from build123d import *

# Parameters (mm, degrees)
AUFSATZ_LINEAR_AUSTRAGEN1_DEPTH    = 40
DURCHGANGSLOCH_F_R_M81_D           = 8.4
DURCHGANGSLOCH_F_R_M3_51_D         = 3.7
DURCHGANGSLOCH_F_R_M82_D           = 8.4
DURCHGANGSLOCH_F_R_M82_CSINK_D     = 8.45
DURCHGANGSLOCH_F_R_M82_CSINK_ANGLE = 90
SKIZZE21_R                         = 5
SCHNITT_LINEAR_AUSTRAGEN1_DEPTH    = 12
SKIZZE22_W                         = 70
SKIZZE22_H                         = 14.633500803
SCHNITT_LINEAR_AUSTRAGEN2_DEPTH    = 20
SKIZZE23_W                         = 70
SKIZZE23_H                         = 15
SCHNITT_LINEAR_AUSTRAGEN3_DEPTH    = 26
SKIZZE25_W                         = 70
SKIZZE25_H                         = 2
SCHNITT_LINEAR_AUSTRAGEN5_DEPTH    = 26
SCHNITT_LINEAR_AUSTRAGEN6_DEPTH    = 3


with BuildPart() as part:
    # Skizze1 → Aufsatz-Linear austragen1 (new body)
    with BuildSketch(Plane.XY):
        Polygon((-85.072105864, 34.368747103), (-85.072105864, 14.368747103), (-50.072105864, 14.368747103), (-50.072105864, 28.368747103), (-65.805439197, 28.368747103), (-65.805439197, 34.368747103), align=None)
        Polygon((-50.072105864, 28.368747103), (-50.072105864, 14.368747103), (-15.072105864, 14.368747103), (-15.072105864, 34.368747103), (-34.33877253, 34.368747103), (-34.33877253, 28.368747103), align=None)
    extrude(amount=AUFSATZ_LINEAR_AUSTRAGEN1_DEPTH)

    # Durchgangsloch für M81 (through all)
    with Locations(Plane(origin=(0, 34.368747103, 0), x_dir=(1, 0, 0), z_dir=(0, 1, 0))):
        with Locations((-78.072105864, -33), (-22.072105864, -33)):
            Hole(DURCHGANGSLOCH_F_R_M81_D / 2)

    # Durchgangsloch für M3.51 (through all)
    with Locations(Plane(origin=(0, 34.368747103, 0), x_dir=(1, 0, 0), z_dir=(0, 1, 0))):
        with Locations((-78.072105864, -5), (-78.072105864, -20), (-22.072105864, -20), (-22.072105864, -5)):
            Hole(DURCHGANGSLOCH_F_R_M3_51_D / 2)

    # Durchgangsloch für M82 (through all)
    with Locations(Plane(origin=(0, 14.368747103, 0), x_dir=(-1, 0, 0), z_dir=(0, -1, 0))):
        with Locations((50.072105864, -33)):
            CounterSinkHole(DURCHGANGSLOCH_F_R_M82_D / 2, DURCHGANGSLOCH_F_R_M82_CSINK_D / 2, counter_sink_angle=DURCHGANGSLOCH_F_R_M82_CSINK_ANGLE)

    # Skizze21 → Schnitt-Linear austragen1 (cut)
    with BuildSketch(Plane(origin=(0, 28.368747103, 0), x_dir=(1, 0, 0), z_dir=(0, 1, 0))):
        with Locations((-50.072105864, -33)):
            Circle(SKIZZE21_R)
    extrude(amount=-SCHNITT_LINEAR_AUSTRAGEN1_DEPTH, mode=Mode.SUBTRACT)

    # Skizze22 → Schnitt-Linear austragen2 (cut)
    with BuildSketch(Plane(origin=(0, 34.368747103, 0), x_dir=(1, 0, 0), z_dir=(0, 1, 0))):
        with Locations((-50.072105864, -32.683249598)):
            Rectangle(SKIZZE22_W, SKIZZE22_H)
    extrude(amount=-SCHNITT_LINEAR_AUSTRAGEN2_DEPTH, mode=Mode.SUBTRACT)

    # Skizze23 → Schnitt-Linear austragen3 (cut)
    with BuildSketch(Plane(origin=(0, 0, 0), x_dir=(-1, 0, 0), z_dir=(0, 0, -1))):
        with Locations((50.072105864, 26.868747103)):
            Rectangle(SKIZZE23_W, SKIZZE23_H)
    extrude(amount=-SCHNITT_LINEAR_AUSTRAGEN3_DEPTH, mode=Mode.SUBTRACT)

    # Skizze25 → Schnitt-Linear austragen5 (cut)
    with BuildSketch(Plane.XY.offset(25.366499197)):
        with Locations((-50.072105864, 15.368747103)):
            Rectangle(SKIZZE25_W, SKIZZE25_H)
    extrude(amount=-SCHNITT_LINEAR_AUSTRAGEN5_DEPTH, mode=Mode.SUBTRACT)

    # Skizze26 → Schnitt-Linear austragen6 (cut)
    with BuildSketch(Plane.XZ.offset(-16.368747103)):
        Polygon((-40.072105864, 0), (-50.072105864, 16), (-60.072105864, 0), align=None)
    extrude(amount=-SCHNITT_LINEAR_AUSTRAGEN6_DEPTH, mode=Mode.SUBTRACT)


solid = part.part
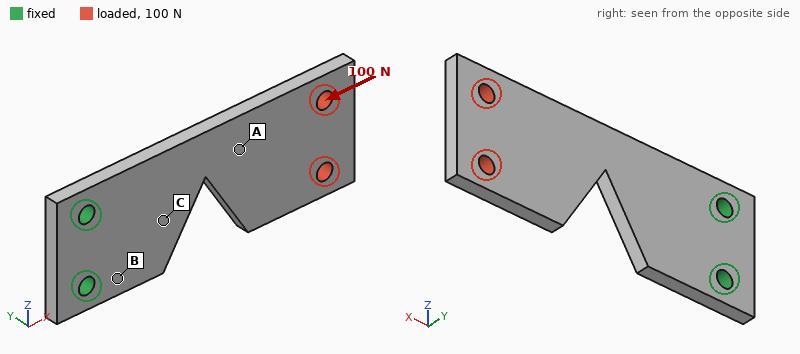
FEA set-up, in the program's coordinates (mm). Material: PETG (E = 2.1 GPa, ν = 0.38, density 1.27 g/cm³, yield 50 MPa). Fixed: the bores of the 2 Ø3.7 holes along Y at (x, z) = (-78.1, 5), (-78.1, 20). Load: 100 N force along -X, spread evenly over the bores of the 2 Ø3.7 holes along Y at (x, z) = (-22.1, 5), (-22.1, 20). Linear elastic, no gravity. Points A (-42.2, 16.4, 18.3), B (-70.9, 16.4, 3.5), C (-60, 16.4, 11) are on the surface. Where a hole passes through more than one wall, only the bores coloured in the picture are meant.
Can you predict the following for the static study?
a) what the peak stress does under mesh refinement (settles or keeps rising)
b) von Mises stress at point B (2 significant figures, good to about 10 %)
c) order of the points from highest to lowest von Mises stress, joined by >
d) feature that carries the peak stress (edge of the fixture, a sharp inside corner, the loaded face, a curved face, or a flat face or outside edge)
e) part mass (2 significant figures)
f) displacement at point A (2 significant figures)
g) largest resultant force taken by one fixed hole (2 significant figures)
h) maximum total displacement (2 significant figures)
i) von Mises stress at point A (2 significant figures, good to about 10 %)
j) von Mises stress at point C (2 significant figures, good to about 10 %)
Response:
keeps rising
1.4 MPa
A > C > B
a sharp inside corner
6.0 g
0.16 mm
51 N
0.79 mm
4.6 MPa
2.9 MPa
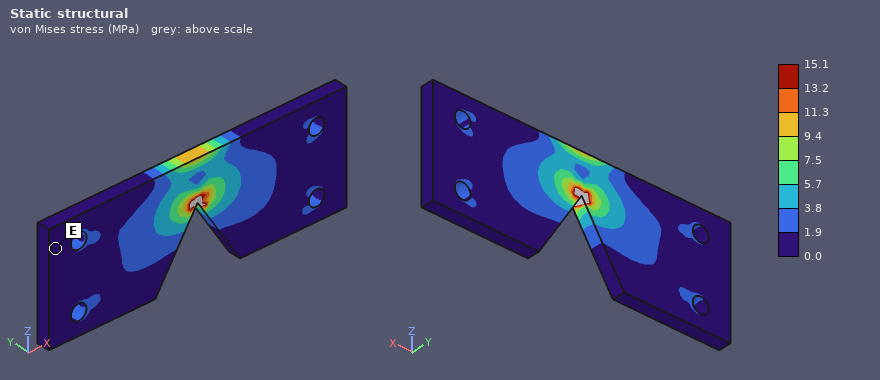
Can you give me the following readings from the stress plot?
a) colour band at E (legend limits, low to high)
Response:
0.0 to 1.9 MPa
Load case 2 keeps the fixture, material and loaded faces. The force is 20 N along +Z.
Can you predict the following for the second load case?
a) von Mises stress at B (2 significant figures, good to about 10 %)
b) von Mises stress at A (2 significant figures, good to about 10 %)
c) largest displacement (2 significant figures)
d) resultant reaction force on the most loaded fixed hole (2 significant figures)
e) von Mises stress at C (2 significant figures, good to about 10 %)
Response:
2.2 MPa
2.5 MPa
0.75 mm
67 N
2.5 MPa
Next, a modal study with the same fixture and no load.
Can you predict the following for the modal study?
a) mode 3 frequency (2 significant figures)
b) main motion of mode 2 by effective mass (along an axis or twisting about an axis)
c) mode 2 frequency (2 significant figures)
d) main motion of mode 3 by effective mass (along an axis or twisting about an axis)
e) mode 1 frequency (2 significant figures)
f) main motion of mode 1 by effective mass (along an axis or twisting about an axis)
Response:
680 Hz
twisting about X
640 Hz
along Z
150 Hz
along Y
